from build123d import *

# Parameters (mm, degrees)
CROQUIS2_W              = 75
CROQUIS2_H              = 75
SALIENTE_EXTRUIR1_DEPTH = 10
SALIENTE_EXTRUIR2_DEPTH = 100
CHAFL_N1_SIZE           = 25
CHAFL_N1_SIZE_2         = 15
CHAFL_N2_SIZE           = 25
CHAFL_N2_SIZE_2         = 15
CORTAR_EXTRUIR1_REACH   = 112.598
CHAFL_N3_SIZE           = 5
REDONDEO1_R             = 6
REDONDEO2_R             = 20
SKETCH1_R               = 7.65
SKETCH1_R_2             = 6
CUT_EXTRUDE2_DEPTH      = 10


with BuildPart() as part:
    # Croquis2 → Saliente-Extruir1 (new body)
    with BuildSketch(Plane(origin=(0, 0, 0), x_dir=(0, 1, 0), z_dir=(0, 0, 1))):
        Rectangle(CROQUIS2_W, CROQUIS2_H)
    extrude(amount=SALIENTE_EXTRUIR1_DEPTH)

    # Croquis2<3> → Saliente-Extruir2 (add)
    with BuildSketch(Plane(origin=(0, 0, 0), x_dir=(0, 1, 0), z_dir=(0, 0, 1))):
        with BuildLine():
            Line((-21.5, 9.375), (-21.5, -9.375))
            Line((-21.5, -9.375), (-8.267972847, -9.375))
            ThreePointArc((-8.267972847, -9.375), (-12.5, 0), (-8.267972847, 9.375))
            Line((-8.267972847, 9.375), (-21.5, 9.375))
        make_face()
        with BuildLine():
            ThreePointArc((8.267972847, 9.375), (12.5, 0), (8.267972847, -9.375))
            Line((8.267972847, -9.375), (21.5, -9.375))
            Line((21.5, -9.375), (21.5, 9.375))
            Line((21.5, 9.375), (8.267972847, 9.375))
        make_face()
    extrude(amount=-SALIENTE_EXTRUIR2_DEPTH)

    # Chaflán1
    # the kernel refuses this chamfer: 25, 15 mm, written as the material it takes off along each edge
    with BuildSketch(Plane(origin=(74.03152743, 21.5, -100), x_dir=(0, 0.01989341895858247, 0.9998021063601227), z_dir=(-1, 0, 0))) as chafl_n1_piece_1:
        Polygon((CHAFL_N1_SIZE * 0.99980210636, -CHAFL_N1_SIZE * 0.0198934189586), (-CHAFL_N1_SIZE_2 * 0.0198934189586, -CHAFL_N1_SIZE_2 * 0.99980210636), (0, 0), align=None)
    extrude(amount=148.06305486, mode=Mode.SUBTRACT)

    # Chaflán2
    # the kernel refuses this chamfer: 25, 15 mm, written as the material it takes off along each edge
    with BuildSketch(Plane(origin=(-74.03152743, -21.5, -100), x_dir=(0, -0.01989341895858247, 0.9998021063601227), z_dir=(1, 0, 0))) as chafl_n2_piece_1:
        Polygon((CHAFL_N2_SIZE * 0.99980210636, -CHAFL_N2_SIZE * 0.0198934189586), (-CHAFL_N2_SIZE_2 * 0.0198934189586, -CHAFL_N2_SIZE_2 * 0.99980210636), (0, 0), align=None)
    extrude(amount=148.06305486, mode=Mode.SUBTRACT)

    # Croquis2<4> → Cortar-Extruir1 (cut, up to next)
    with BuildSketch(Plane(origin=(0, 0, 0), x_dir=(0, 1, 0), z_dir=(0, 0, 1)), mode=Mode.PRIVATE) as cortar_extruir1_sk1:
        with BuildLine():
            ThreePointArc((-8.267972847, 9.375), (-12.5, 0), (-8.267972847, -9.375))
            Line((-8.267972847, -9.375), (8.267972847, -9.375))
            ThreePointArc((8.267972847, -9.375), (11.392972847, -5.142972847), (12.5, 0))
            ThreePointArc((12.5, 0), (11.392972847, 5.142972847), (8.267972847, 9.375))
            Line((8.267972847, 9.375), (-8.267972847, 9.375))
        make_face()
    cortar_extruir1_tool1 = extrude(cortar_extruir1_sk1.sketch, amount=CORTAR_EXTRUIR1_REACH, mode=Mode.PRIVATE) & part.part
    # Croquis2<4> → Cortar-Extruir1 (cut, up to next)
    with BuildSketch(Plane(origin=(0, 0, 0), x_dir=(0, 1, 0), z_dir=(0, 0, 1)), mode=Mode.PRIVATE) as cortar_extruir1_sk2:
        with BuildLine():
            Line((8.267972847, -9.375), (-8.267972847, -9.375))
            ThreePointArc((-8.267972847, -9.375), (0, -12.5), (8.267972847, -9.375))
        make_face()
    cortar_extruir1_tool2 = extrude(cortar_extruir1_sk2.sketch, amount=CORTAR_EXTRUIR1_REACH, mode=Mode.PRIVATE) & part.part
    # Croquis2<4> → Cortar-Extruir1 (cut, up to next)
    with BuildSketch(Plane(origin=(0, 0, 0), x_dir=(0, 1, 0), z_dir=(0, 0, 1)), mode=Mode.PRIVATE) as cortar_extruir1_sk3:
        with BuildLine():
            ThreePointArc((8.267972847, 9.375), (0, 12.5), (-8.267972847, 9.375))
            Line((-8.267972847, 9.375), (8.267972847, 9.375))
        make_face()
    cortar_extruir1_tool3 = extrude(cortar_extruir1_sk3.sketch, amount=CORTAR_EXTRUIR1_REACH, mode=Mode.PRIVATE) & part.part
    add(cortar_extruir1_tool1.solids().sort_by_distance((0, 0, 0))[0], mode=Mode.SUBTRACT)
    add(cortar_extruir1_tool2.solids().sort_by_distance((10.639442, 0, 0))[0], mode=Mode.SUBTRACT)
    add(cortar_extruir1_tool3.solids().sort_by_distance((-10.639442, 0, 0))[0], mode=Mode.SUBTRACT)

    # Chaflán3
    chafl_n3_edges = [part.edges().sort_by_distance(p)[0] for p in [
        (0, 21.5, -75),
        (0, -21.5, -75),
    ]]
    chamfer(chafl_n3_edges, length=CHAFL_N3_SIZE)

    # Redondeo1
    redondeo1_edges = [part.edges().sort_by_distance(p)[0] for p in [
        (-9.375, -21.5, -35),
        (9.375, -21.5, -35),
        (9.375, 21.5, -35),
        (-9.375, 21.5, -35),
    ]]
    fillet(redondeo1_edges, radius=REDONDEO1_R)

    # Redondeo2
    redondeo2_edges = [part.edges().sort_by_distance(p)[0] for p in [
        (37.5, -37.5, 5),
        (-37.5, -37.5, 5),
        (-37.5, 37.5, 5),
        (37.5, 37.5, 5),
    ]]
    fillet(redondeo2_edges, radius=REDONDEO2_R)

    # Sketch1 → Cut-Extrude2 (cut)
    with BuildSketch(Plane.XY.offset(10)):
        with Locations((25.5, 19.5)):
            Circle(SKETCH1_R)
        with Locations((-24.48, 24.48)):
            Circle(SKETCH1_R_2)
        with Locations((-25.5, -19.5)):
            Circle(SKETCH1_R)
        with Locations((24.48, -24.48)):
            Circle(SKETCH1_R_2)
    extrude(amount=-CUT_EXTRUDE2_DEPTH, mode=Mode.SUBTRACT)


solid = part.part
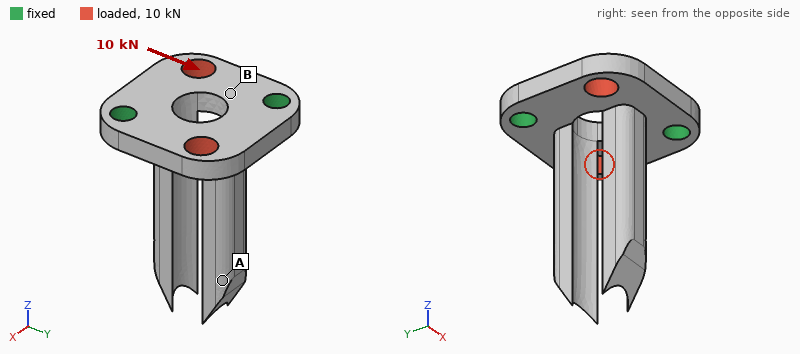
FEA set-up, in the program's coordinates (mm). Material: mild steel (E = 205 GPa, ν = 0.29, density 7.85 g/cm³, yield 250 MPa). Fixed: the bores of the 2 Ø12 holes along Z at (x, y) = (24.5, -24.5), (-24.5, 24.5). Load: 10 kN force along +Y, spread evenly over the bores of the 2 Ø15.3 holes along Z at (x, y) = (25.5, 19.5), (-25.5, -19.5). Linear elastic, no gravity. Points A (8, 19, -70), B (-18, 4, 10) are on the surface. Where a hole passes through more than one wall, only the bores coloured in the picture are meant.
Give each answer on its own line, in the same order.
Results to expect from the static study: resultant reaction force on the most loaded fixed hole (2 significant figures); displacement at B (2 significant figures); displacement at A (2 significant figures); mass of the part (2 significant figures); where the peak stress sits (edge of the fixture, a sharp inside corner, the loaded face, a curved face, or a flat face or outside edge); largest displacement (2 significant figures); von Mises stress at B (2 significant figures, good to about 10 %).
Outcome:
5.0 kN
1.8 µm
2.8 µm
560 g
the loaded face
7.1 µm
17 MPa
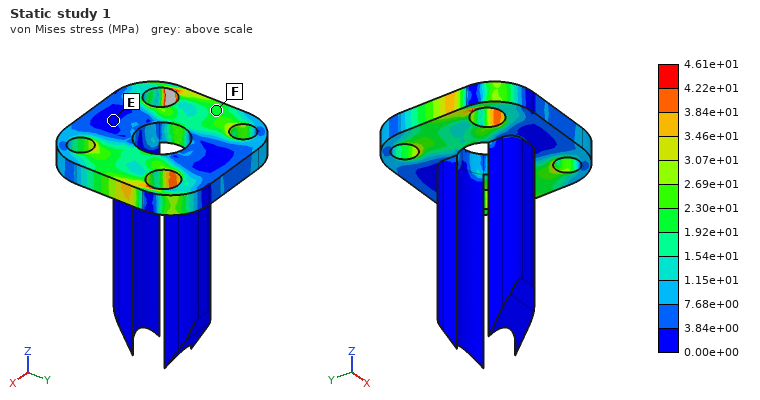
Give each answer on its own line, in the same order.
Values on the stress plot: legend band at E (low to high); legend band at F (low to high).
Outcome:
0.00e+00 to 3.84e+00 MPa
1.92e+01 to 2.30e+01 MPa
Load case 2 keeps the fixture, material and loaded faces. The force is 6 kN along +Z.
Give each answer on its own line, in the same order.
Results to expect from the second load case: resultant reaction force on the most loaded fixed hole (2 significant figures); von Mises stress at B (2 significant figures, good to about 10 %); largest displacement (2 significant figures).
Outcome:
3.0 kN
66 MPa
90 µm
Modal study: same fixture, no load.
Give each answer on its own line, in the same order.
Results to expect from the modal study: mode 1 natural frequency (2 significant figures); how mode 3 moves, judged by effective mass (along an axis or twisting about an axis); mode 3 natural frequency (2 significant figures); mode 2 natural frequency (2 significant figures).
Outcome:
1000 Hz
along X
1500 Hz
1000 Hz
